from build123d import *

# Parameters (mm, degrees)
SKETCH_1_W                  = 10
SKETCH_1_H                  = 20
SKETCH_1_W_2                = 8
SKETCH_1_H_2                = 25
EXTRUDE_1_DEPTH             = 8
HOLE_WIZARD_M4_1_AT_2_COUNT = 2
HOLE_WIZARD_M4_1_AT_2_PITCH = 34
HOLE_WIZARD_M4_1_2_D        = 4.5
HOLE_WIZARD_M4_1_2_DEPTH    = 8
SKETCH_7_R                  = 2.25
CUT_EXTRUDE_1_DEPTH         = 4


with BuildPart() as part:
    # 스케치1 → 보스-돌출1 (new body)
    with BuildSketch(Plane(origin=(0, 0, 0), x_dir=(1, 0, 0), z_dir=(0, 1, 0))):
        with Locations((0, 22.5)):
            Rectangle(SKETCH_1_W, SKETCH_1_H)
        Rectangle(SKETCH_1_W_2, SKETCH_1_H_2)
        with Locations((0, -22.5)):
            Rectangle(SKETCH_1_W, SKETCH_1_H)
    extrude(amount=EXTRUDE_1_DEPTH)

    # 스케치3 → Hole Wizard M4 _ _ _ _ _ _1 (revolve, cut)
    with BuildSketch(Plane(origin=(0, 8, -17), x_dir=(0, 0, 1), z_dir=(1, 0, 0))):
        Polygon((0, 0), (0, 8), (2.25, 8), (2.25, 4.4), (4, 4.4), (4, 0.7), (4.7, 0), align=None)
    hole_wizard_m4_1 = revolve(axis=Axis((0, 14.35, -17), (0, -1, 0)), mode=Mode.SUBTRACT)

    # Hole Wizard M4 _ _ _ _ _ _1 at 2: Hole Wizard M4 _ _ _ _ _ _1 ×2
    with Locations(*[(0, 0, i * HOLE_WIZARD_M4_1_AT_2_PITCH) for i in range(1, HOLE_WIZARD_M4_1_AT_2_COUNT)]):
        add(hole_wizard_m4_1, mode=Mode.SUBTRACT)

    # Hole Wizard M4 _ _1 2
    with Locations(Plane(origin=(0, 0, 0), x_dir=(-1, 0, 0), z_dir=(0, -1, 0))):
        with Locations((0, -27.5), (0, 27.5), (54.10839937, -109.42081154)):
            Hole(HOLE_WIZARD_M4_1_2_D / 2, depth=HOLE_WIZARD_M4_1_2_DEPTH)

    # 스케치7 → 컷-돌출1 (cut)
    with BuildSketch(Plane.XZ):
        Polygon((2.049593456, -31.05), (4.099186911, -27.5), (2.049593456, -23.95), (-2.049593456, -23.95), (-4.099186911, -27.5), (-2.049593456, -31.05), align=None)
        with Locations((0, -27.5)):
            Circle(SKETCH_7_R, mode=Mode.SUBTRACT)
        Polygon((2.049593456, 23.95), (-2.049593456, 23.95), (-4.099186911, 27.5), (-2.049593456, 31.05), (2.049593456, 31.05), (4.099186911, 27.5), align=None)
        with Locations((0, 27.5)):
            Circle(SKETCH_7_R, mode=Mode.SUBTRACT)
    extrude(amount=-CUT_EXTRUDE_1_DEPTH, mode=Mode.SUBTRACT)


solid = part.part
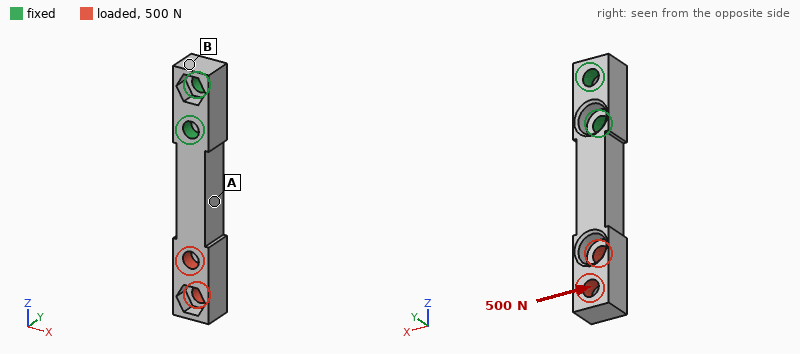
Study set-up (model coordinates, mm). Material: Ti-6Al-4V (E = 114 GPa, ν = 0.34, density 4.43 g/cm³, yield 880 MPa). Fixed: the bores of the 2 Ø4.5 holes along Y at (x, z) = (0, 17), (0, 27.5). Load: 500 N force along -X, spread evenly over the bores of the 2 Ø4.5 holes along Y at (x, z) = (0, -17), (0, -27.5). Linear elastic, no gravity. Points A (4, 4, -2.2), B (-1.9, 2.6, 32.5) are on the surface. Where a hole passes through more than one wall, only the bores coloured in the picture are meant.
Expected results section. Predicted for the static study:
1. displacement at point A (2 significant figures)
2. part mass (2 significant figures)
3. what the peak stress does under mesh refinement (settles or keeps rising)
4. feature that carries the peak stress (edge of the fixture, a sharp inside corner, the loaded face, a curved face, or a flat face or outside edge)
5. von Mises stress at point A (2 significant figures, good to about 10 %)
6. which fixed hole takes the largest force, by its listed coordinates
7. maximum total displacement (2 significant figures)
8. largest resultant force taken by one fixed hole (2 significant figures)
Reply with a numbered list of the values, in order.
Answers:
1. 0.099 mm
2. 17 g
3. keeps rising
4. edge of the fixture
5. 120 MPa
6. (0, 17)
7. 0.43 mm
8. 1.0 kN
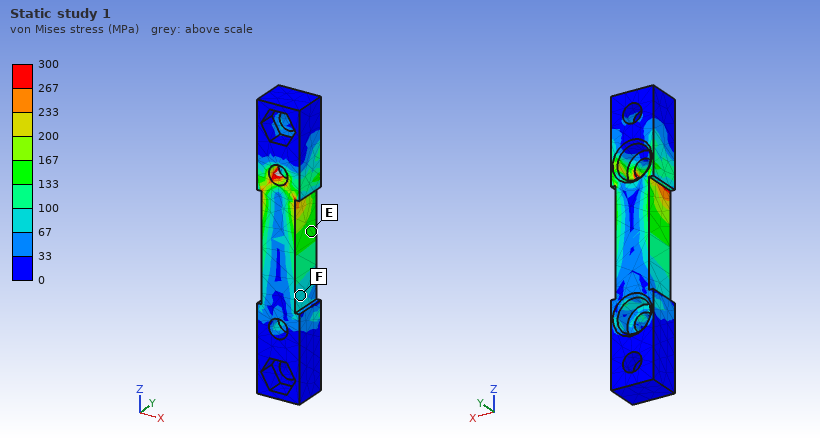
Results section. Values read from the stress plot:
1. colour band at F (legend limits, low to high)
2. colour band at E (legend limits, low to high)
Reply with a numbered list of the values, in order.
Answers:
1. 67 to 100 MPa
2. 133 to 167 MPa
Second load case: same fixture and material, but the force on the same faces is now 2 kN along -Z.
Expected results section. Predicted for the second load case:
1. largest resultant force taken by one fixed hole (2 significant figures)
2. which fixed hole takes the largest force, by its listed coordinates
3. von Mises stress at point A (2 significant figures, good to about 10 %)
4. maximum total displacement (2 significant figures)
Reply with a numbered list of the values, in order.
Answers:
1. 1.6 kN
2. (0, 17)
3. 31 MPa
4. 99 µm
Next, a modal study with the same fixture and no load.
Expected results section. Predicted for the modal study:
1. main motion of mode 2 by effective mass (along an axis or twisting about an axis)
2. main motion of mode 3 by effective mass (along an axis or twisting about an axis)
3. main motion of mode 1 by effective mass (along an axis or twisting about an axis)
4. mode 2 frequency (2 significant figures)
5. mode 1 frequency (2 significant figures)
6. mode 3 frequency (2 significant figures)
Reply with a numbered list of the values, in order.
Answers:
1. along X
2. twisting about Z
3. along Y
4. 2600 Hz
5. 2200 Hz
6. 12 kHz
